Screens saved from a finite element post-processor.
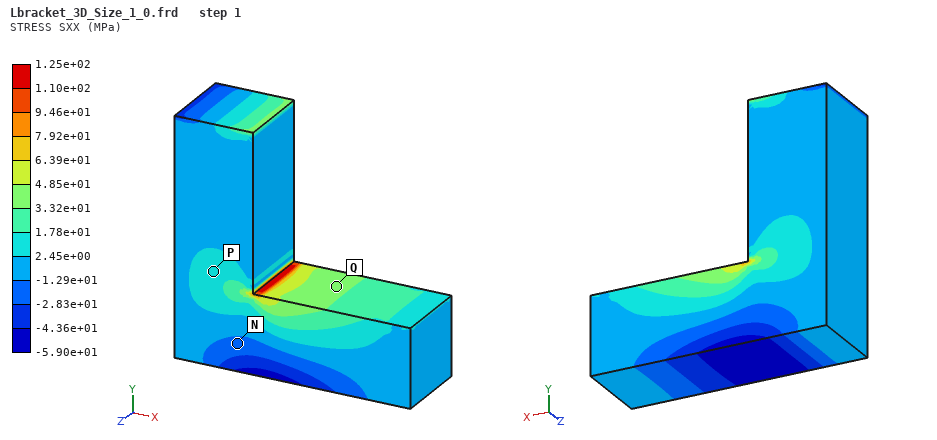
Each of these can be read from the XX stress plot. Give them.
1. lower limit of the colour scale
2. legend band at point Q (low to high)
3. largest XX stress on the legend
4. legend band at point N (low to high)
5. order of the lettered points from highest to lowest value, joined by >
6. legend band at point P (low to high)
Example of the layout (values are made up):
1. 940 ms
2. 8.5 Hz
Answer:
1. -5.90e+01 MPa
2. 3.32e+01 to 4.85e+01 MPa
3. 1.25e+02 MPa
4. -2.83e+01 to -1.29e+01 MPa
5. Q > P > N
6. 2.45e+00 to 1.78e+01 MPa
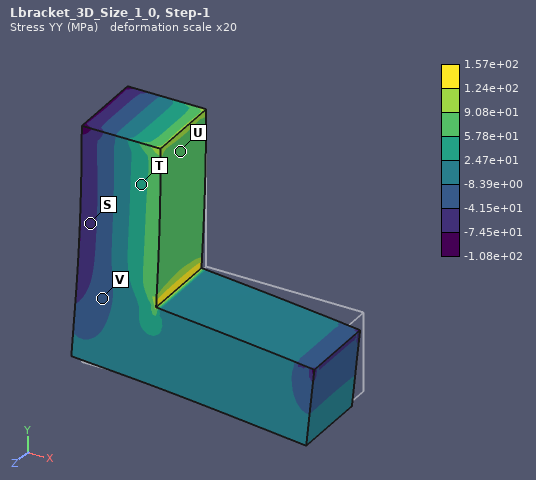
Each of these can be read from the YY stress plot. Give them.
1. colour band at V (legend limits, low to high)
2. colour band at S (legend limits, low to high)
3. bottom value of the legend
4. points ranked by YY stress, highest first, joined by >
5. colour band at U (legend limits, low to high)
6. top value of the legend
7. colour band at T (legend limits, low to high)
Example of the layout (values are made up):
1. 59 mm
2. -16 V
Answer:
1. -4.15e+01 to -8.39e+00 MPa
2. -7.45e+01 to -4.15e+01 MPa
3. -1.08e+02 MPa
4. U > T > V > S
5. 5.78e+01 to 9.08e+01 MPa
6. 1.57e+02 MPa
7. 2.47e+01 to 5.78e+01 MPa
